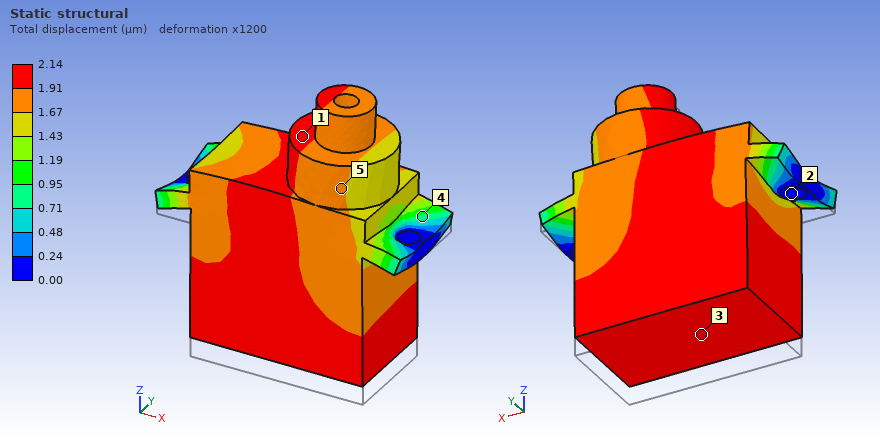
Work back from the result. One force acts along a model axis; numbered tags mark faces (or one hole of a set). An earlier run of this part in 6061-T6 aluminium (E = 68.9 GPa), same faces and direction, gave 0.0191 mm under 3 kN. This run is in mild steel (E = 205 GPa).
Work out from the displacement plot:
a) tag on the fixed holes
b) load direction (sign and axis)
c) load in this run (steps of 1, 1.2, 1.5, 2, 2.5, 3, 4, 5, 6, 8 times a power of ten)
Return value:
2
+Z
1 kN
